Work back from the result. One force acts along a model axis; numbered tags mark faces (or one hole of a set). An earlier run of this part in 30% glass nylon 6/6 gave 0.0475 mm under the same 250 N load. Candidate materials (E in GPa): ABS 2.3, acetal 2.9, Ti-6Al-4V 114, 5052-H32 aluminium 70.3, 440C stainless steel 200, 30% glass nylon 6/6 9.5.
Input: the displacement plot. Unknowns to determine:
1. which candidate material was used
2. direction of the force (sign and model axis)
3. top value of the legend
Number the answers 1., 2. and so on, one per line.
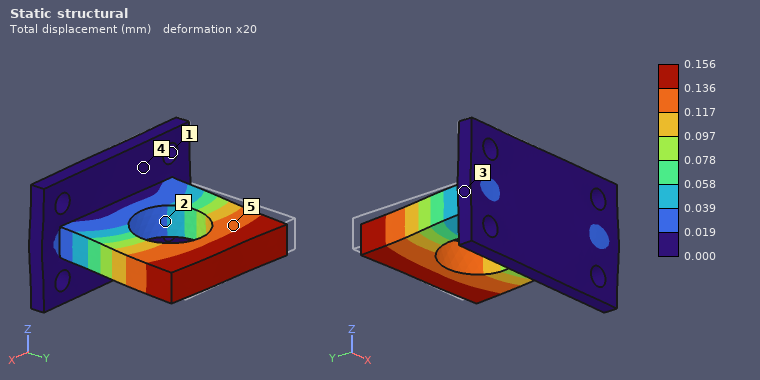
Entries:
1. acetal
2. +X
3. 0.156 mm
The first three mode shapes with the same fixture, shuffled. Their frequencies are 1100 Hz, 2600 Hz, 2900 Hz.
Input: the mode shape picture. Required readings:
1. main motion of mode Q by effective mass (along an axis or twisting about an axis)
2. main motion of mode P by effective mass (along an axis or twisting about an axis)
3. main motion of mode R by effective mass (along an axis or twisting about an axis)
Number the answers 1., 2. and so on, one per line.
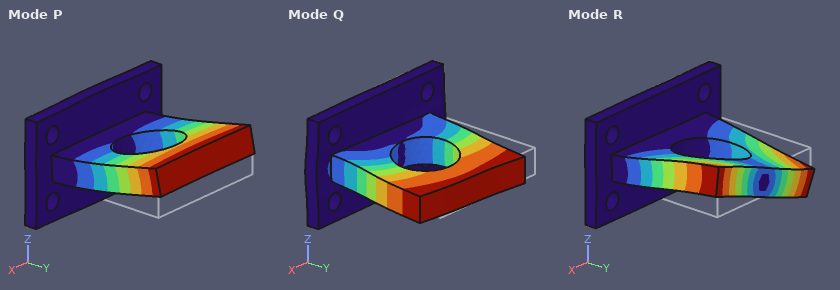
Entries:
1. along X
2. along Z
3. twisting about Y
